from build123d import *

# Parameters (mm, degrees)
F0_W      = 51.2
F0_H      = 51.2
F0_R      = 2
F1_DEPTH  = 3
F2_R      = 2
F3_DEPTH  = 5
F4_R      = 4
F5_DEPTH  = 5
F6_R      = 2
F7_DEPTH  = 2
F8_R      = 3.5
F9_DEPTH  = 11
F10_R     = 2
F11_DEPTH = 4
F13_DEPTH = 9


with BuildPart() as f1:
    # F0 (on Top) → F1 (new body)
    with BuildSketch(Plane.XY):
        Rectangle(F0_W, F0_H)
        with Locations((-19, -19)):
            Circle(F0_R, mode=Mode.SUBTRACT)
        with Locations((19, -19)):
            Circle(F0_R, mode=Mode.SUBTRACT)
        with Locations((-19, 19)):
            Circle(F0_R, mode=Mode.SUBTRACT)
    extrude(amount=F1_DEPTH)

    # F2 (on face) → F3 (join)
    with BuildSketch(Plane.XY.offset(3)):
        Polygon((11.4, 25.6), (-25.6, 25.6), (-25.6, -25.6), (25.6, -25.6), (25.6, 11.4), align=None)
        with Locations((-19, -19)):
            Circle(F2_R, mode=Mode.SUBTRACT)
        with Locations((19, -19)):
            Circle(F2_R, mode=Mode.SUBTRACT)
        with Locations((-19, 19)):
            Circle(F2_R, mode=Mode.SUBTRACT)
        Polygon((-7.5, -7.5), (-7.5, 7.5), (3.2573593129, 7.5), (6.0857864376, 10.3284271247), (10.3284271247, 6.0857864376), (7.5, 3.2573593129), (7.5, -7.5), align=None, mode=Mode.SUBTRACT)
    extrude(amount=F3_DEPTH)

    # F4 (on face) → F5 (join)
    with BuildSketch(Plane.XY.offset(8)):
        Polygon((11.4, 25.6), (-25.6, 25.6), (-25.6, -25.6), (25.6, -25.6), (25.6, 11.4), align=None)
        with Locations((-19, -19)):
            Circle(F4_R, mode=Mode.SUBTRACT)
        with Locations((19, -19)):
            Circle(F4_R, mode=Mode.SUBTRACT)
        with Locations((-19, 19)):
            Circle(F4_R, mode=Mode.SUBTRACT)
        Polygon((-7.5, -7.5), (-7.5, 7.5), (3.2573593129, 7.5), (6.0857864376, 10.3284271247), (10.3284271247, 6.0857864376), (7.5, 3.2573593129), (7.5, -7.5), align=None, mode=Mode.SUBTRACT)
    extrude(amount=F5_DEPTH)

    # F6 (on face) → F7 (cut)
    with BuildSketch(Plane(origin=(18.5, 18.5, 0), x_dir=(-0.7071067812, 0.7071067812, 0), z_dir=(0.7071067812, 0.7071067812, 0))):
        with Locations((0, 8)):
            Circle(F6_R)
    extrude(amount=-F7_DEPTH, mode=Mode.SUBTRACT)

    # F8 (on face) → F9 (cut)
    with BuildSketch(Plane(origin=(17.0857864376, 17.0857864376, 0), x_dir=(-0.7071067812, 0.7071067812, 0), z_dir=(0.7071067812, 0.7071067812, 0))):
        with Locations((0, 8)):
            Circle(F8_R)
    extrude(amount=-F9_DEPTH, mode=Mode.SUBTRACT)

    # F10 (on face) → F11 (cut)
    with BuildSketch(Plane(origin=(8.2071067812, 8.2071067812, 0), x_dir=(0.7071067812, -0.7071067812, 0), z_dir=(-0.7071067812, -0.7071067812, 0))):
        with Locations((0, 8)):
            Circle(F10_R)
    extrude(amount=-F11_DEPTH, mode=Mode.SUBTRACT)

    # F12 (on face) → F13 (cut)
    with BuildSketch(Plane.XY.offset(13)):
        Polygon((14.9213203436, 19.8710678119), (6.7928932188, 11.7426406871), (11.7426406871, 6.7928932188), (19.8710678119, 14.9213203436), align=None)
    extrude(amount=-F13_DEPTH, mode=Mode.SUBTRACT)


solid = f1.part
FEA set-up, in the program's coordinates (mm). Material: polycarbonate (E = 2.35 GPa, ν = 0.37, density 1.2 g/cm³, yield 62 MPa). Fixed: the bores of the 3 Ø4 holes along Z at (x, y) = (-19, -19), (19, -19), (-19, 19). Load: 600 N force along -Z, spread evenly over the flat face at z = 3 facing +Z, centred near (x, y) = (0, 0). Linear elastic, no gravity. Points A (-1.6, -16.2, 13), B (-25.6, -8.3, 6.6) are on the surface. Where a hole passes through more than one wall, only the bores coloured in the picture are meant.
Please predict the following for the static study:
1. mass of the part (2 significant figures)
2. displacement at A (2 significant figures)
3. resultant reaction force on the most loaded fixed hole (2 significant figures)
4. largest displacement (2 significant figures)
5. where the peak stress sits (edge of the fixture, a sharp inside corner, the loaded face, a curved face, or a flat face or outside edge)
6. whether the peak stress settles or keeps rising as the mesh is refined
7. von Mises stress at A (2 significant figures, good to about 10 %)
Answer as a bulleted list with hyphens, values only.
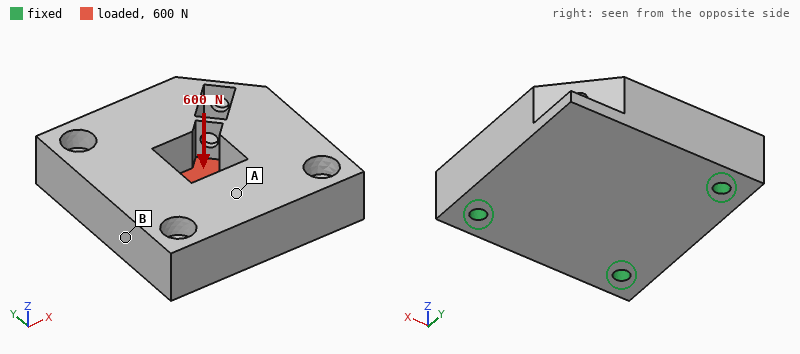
- 35 g
- 0.049 mm
- 250 N
- 0.24 mm
- edge of the fixture
- keeps rising
- 3.9 MPa
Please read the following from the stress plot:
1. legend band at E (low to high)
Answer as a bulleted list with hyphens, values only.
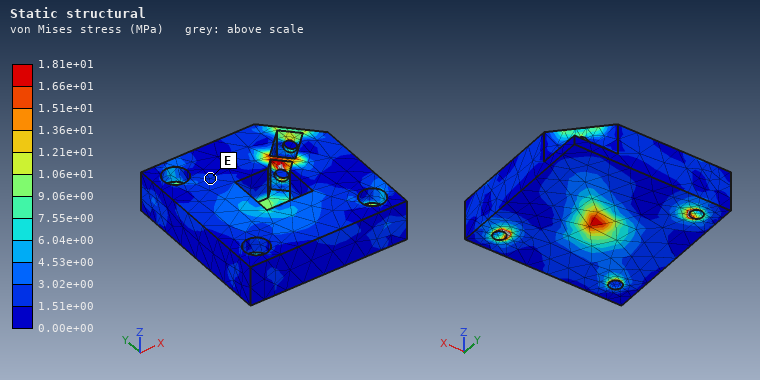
- 1.51e+00 to 3.02e+00 MPa
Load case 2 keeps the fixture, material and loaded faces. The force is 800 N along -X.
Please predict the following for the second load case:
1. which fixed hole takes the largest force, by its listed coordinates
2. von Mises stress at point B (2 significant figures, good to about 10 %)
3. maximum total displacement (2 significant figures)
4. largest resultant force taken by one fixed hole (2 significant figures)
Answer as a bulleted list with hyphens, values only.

- (-19, 19)
- 1.1 MPa
- 56 µm
- 340 N
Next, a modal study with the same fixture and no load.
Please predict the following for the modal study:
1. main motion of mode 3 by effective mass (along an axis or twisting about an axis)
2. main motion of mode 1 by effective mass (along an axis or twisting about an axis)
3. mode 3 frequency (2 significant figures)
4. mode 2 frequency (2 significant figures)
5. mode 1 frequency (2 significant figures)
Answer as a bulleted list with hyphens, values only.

- along Z
- along Z
- 5500 Hz
- 5100 Hz
- 2100 Hz
